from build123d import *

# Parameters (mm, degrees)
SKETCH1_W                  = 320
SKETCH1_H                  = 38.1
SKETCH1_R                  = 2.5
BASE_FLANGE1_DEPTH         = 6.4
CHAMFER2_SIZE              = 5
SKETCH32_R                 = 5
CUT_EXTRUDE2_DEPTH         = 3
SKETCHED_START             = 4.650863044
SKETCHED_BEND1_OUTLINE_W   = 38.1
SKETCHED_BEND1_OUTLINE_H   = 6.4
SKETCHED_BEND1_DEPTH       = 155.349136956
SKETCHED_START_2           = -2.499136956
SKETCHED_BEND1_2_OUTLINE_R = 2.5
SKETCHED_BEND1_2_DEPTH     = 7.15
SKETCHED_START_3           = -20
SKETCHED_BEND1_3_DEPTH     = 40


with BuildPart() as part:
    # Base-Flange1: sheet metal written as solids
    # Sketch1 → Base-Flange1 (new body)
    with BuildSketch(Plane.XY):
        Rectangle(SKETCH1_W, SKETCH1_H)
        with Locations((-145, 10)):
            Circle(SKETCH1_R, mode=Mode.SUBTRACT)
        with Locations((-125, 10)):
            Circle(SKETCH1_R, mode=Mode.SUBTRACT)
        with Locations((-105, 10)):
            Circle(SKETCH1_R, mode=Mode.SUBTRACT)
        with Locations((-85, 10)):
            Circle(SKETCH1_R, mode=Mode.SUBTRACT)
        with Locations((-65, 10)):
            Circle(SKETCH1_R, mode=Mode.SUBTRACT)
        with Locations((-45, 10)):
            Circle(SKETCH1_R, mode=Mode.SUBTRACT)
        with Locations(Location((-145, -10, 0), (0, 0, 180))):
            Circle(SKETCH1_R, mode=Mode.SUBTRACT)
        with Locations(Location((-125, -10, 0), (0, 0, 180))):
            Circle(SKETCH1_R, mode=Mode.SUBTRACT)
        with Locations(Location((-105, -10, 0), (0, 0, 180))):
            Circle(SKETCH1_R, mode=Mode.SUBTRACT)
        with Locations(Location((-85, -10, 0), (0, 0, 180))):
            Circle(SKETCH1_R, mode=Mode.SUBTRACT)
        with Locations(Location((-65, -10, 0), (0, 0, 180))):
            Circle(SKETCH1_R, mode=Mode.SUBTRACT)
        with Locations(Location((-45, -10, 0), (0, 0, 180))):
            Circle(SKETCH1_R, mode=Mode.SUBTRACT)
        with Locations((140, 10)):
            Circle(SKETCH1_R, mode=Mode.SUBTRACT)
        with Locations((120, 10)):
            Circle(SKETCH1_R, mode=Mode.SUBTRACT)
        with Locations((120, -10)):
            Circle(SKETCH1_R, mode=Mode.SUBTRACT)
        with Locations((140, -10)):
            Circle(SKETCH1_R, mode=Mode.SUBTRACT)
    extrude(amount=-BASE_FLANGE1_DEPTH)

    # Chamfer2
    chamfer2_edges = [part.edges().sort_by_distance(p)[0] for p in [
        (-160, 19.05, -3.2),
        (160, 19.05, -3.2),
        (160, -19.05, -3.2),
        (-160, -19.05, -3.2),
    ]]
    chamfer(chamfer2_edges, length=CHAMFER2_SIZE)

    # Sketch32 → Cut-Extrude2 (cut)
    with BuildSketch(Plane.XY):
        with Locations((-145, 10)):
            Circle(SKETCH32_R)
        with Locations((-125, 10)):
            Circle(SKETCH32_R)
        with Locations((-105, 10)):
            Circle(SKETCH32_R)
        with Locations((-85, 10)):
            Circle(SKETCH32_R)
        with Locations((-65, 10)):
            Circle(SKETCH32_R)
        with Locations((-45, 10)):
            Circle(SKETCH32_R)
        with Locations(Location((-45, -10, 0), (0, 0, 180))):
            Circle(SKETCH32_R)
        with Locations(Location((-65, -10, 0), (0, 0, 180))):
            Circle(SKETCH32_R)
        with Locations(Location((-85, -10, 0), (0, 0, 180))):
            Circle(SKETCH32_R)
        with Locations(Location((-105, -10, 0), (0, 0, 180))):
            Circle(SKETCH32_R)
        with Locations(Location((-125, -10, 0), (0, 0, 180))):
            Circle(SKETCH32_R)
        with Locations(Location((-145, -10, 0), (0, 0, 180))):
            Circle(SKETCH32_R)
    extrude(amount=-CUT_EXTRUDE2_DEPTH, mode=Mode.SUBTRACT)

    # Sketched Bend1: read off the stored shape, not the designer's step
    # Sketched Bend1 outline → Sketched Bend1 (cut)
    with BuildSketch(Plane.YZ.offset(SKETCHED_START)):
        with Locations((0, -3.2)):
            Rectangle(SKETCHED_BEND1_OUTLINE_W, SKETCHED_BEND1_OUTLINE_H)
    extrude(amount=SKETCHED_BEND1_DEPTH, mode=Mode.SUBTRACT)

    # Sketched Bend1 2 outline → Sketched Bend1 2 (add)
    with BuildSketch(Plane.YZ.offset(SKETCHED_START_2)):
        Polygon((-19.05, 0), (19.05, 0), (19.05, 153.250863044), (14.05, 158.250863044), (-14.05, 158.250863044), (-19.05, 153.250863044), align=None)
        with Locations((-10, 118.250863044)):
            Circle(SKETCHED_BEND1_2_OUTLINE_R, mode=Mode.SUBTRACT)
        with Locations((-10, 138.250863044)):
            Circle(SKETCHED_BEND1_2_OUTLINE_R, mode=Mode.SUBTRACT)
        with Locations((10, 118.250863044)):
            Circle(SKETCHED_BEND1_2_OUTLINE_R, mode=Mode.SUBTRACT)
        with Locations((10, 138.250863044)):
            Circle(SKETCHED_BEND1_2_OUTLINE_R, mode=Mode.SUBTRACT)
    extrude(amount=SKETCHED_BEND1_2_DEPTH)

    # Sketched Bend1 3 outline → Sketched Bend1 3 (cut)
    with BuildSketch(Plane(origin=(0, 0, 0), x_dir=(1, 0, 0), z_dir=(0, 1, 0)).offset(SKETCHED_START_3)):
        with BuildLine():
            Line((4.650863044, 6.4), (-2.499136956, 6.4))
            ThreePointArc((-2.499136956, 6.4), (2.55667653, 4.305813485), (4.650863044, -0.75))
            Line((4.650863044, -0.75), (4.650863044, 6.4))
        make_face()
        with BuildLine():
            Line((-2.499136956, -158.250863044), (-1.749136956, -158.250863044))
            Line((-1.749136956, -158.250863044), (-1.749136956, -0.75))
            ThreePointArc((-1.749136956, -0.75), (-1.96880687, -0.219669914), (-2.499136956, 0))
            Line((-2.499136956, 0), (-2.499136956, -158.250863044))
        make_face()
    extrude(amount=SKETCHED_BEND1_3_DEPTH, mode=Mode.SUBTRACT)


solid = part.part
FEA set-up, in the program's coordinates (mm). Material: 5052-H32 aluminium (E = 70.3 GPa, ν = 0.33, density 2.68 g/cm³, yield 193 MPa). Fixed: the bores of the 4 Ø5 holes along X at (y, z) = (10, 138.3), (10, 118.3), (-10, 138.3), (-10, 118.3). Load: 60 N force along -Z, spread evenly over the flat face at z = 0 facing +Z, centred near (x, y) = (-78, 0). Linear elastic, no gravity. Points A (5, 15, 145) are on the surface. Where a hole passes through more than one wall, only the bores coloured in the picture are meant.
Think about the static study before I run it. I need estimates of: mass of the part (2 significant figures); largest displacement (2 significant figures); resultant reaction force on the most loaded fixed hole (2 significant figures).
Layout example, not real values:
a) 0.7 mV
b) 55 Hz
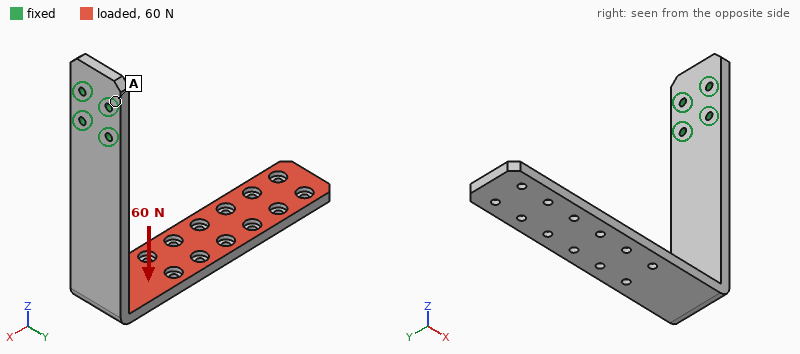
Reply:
a) 200 g
b) 2.2 mm
c) 37 N
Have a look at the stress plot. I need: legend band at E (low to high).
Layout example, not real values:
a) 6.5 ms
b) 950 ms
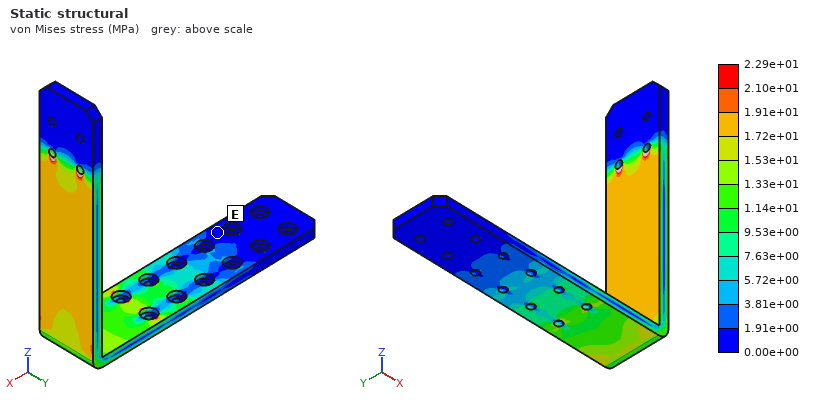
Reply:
a) 0.00e+00 to 1.91e+00 MPa
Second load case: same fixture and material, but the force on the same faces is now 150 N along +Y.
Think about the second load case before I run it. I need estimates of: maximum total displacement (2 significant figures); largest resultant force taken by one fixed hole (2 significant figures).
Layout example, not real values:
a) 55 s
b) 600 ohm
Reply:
a) 2.7 mm
b) 800 N
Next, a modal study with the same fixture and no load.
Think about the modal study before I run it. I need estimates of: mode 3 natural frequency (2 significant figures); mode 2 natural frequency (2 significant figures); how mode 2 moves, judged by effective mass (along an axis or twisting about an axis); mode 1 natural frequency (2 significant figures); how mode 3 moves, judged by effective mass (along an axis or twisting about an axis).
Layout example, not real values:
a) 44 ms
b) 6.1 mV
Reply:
a) 250 Hz
b) 150 Hz
c) along Y
d) 93 Hz
e) along X
